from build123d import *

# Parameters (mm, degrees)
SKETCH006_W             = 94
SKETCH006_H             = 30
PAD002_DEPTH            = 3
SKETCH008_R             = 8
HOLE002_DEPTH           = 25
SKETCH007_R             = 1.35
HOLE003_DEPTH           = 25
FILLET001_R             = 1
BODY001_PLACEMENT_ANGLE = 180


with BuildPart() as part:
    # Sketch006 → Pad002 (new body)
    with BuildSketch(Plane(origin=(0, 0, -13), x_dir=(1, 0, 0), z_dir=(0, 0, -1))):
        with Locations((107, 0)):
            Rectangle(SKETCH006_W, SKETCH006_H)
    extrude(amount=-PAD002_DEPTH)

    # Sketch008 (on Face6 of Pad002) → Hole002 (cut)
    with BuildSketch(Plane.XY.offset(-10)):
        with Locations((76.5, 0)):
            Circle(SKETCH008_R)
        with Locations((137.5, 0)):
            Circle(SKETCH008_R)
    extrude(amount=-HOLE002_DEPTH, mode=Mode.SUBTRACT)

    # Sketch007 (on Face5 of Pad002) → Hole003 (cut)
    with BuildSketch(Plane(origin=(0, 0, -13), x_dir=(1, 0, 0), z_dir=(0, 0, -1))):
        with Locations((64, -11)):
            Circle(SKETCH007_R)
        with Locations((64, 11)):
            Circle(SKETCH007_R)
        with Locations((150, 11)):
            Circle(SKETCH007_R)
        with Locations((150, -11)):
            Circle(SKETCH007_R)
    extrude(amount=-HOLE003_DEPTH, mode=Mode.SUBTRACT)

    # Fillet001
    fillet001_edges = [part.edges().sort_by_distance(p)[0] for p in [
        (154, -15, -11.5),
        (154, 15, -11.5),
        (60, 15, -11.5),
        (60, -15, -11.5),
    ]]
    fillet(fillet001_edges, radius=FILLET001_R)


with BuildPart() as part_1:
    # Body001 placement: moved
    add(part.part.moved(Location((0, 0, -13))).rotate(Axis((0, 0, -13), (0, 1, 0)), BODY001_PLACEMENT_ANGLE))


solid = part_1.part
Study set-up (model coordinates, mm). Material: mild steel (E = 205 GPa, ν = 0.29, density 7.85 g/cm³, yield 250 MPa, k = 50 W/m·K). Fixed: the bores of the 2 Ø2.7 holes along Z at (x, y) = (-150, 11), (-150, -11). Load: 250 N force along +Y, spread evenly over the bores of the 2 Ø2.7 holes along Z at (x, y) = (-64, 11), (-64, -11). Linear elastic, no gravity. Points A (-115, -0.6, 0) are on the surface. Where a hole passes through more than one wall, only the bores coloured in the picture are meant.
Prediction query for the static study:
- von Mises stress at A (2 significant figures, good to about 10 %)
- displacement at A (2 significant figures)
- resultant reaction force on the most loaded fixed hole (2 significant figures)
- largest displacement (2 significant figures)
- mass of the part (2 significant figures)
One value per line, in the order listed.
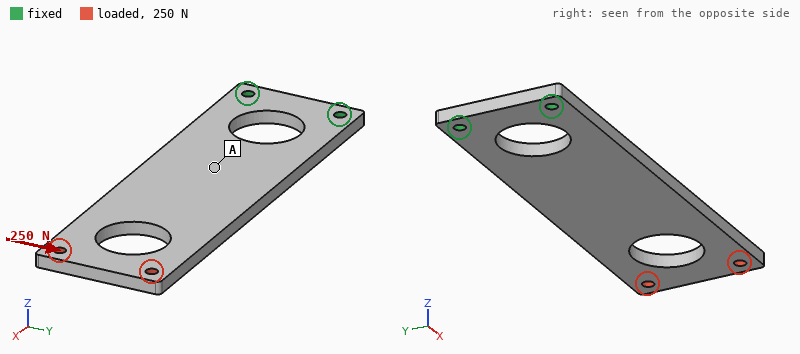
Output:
7.6 MPa
14 µm
920 N
56 µm
56 g
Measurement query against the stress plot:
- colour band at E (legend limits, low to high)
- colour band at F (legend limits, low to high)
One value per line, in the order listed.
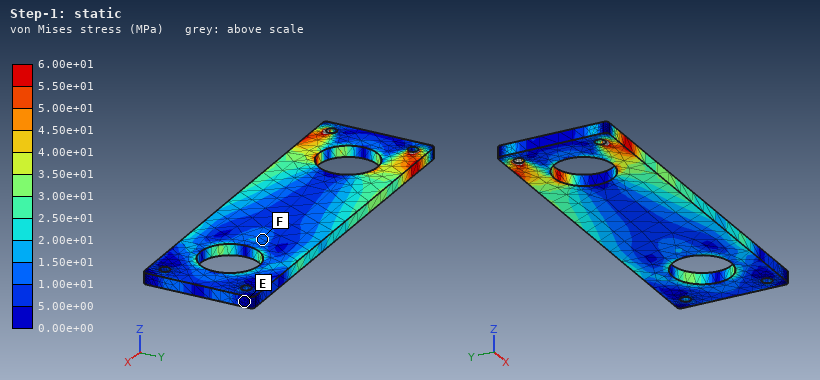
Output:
0.00e+00 to 5.00e+00 MPa
1.00e+01 to 1.50e+01 MPa
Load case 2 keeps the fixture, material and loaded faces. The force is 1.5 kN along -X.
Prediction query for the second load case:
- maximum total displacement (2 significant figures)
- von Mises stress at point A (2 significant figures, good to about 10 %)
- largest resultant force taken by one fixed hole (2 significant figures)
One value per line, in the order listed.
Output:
12 µm
12 MPa
750 N
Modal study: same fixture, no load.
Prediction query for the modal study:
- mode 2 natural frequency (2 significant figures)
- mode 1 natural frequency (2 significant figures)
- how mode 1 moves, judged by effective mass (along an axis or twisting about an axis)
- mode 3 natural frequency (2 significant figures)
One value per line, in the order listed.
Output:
1700 Hz
270 Hz
along Z
1800 Hz
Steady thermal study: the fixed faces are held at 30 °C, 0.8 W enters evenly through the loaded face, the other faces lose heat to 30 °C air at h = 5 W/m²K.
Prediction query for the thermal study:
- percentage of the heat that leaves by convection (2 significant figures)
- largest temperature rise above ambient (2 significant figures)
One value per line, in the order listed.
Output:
30 %
18 K
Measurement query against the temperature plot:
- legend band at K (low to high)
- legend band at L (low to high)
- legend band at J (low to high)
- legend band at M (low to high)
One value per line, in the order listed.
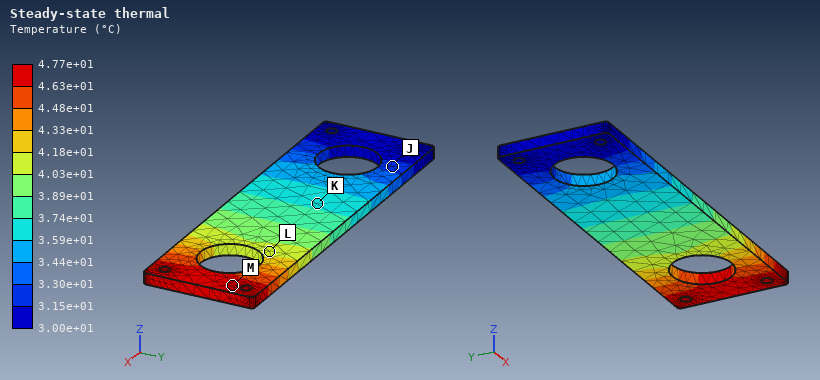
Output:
3.59e+01 to 3.74e+01 °C
4.03e+01 to 4.18e+01 °C
3.15e+01 to 3.30e+01 °C
4.63e+01 to 4.77e+01 °C
